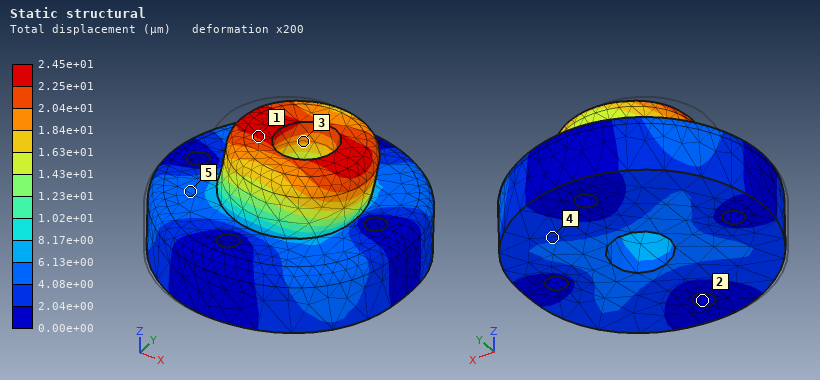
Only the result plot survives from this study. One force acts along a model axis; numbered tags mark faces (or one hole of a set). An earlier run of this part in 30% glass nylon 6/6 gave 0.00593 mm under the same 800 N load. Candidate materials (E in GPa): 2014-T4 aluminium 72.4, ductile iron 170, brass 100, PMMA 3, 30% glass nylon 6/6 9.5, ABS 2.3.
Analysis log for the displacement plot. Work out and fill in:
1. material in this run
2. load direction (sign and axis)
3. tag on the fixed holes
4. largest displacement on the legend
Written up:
ABS
+X
2
2.45e+01 µm
